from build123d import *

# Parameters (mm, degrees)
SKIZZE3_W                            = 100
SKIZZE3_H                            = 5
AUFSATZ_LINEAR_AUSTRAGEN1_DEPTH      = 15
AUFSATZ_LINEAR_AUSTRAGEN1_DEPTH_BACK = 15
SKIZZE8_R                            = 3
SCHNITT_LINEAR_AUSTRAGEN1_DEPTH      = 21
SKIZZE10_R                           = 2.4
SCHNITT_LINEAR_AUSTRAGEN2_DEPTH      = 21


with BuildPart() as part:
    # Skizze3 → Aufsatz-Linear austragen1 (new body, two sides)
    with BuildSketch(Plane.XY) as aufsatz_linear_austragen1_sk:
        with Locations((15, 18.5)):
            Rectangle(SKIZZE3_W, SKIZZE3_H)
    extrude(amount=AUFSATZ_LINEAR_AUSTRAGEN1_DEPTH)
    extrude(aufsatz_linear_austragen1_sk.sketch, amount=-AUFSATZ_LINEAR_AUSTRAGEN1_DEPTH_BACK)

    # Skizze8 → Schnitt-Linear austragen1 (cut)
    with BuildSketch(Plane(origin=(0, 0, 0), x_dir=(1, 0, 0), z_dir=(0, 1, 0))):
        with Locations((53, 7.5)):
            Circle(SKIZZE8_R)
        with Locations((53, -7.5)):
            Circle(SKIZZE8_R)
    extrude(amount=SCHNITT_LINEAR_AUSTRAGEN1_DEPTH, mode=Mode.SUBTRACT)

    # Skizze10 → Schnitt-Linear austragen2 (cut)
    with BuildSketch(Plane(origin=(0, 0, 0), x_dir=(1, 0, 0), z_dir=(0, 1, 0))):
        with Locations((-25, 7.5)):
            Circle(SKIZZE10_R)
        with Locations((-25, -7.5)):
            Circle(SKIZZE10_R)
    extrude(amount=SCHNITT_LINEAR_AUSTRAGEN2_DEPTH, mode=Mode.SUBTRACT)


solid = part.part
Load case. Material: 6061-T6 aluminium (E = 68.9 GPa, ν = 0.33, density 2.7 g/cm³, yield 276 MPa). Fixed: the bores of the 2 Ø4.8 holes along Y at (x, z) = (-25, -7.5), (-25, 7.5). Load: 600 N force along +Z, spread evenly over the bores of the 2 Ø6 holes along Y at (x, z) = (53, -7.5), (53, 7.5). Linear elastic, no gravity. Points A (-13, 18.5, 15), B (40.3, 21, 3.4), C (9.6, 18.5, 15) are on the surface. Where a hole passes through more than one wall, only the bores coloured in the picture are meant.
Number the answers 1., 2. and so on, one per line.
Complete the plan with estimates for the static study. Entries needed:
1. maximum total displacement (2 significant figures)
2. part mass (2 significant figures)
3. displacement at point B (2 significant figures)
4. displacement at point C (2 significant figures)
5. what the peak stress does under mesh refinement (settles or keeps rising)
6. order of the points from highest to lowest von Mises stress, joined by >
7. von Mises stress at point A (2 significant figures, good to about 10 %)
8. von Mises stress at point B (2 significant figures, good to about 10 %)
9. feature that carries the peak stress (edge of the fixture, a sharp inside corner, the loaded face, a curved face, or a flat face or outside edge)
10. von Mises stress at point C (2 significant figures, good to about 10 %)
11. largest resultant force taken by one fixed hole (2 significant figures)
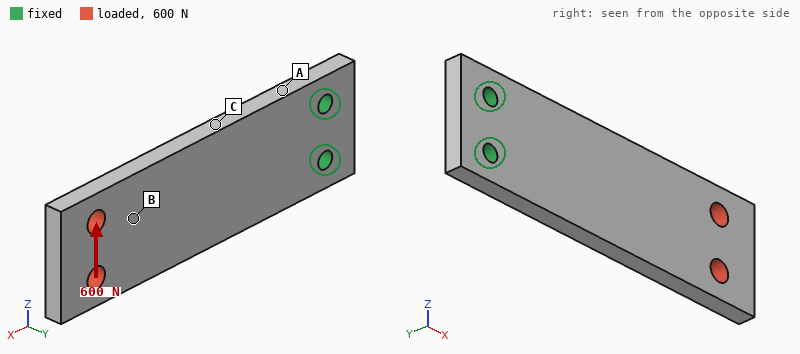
1. 0.18 mm
2. 39 g
3. 0.11 mm
4. 0.051 mm
5. keeps rising
6. A > C > B
7. 49 MPa
8. 10 MPa
9. edge of the fixture
10. 35 MPa
11. 2.6 kN
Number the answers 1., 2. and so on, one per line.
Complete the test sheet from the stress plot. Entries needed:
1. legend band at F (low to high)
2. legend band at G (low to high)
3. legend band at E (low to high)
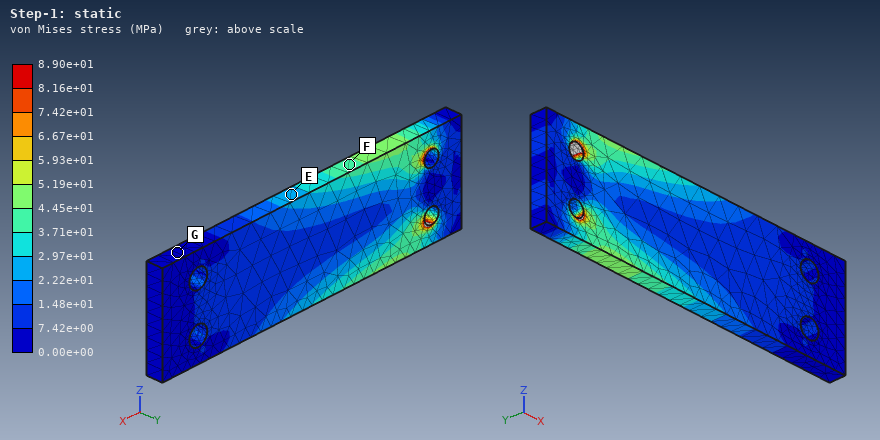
1. 3.71e+01 to 4.45e+01 MPa
2. 0.00e+00 to 7.42e+00 MPa
3. 2.22e+01 to 2.97e+01 MPa
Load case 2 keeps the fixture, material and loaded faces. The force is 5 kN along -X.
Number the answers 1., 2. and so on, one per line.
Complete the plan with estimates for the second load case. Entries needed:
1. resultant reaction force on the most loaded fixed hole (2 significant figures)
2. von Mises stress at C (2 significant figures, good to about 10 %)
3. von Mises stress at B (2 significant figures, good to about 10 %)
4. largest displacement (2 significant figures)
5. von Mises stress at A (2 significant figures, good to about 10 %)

1. 2.5 kN
2. 33 MPa
3. 34 MPa
4. 42 µm
5. 28 MPa
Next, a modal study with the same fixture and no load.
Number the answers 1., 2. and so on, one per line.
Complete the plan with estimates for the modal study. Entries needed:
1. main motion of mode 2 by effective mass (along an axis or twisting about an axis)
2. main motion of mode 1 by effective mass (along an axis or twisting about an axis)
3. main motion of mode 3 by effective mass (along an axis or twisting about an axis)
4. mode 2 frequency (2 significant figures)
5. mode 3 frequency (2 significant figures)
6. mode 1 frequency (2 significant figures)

1. along Z
2. along Y
3. twisting about X
4. 2700 Hz
5. 3000 Hz
6. 530 Hz
